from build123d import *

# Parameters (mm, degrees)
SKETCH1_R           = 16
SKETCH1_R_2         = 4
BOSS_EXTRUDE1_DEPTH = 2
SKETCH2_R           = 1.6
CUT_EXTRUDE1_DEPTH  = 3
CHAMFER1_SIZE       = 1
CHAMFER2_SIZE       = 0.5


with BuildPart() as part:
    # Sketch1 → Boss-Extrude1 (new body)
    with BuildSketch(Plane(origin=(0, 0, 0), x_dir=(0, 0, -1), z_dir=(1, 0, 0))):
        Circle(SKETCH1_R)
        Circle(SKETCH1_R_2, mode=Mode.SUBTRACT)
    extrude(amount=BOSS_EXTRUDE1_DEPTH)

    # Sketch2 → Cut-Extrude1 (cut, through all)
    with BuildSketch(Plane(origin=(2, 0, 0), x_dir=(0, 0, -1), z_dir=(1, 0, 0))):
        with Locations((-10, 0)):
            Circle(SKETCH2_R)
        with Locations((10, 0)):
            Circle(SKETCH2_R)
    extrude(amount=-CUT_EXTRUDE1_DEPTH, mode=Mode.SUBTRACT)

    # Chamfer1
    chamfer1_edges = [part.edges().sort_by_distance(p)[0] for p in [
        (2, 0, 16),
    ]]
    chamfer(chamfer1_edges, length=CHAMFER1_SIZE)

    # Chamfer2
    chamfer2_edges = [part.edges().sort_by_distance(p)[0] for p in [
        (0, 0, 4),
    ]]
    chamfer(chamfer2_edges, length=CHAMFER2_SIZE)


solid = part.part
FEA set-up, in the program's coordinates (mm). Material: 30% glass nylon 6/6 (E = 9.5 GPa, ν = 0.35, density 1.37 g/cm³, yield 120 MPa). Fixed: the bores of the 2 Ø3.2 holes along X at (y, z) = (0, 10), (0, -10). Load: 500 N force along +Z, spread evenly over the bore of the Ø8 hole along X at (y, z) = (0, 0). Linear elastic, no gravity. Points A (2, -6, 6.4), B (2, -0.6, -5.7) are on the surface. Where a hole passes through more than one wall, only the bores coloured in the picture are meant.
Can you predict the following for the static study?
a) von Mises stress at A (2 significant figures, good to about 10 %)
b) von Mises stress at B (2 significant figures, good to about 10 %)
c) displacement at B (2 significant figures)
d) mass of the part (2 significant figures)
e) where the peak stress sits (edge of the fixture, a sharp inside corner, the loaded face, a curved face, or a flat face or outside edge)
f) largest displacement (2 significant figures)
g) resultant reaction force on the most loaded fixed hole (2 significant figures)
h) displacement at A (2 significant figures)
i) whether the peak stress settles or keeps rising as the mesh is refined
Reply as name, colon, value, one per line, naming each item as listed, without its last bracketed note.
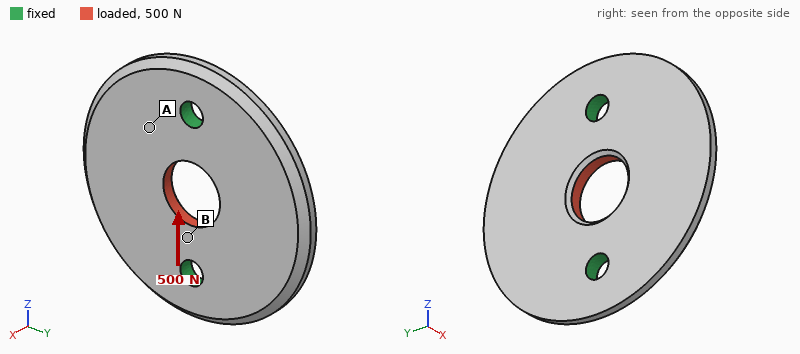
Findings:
von Mises stress at A: 4.3 MPa
von Mises stress at B: 18 MPa
displacement at B: 5.8 µm
mass of the part: 1.9 g
where the peak stress sits: edge of the fixture
largest displacement: 13 µm
resultant reaction force on the most loaded fixed hole: 250 N
displacement at A: 7.7 µm
whether the peak stress settles or keeps rising as the mesh is refined: keeps rising
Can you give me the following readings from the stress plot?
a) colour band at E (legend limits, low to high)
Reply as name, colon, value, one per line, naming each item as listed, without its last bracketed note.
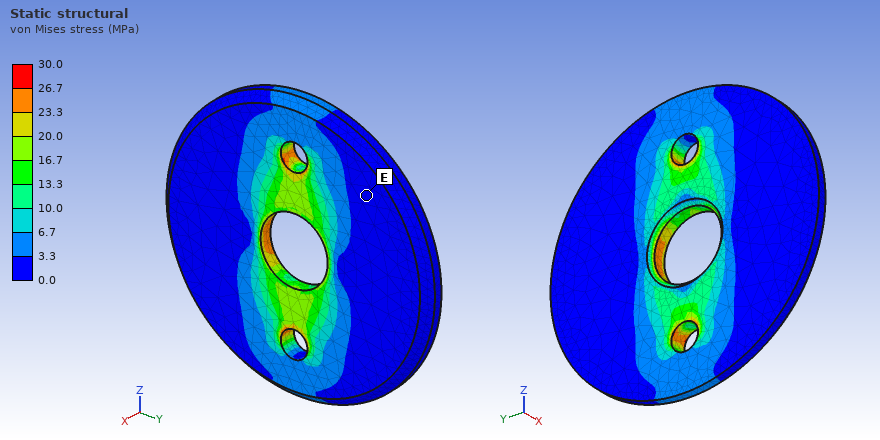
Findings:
colour band at E: 0.0 to 3.3 MPa
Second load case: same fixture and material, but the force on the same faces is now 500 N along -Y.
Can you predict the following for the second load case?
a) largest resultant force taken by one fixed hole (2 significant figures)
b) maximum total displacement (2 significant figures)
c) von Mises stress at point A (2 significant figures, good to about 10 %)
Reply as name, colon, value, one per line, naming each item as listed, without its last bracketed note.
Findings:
largest resultant force taken by one fixed hole: 250 N
maximum total displacement: 29 µm
von Mises stress at point A: 9.1 MPa
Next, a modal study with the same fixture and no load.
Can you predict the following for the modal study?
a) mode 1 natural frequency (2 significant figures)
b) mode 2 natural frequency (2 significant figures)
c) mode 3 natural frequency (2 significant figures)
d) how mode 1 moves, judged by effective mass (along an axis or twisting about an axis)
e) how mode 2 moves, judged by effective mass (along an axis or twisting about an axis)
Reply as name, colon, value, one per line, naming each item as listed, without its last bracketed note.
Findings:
mode 1 natural frequency: 3900 Hz
mode 2 natural frequency: 4200 Hz
mode 3 natural frequency: 9300 Hz
how mode 1 moves, judged by effective mass: twisting about Z
how mode 2 moves, judged by effective mass: along X
